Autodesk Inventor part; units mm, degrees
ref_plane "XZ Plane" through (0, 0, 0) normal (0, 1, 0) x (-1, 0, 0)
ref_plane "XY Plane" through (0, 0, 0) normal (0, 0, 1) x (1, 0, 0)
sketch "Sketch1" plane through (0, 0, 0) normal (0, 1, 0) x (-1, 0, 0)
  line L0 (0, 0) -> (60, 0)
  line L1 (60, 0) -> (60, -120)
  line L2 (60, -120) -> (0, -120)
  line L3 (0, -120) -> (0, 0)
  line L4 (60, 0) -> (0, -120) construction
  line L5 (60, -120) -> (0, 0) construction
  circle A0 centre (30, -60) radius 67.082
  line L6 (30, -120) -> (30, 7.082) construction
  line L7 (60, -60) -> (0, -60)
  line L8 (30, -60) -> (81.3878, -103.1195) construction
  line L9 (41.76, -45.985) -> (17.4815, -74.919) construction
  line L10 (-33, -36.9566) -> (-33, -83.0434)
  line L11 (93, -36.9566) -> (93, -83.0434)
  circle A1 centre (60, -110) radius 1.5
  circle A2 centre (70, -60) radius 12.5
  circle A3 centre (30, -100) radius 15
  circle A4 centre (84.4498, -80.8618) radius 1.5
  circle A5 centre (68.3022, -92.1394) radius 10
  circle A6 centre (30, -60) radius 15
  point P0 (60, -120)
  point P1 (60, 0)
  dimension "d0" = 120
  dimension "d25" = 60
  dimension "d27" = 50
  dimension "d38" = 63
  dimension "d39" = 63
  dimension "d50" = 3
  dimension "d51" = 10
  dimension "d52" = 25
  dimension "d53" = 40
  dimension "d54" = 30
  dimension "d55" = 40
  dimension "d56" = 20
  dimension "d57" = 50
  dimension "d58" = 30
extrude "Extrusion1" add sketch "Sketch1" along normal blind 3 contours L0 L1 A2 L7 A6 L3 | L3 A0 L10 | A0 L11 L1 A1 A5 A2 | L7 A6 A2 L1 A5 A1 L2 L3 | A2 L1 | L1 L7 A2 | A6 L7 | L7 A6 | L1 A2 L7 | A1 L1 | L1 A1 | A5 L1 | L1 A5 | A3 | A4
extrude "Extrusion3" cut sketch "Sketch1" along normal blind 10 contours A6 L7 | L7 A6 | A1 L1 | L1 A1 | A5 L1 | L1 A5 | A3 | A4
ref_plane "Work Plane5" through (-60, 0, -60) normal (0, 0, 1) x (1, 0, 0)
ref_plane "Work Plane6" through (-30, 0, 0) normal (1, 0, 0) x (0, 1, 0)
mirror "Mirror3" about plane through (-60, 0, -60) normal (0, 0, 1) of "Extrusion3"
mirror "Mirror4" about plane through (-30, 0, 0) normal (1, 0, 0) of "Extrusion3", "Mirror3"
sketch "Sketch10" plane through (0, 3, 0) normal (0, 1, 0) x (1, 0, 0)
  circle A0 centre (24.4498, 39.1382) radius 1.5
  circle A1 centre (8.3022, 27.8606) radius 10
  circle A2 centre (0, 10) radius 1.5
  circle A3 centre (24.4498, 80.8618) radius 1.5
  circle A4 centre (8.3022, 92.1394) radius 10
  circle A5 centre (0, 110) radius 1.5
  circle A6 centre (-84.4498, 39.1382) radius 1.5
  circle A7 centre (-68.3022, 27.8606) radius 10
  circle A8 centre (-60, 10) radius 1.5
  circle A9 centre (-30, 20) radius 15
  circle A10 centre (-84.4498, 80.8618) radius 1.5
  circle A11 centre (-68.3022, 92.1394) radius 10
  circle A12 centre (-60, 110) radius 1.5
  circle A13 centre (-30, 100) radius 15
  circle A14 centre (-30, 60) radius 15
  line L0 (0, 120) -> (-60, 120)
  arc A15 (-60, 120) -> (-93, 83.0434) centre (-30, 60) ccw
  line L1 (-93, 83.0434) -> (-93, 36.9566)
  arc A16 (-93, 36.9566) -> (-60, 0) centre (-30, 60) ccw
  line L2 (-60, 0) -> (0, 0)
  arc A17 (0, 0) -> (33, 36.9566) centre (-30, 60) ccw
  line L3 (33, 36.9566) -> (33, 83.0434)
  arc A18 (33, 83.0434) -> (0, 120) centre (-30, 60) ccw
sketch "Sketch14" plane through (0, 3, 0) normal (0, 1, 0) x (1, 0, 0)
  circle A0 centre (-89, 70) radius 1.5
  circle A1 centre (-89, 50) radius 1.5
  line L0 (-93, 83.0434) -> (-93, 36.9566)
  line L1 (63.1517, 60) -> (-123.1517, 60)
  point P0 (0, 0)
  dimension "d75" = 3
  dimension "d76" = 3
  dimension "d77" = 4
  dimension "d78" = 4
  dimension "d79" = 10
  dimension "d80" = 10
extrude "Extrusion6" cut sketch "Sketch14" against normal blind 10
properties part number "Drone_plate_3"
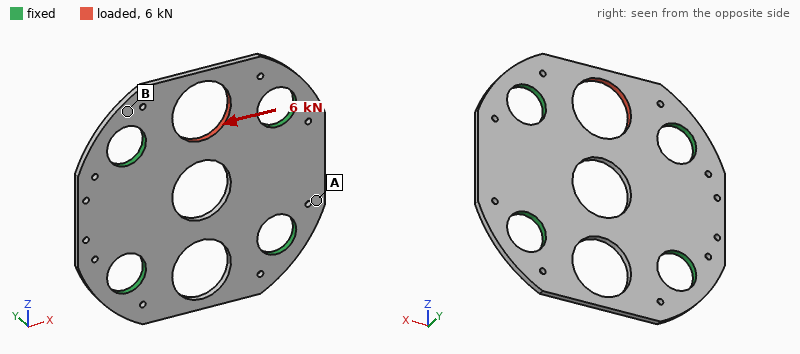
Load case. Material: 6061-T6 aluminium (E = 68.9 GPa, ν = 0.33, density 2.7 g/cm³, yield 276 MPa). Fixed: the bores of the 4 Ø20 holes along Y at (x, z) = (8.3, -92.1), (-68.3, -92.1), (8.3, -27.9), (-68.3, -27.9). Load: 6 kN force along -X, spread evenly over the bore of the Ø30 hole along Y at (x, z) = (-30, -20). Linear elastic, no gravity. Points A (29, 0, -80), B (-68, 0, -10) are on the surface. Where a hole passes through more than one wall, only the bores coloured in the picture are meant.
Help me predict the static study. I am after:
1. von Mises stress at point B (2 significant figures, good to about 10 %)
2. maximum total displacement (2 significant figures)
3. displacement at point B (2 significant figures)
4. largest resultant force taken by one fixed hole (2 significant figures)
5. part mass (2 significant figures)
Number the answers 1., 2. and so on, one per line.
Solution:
1. 23 MPa
2. 25 µm
3. 6.4 µm
4. 2.9 kN
5. 80 g
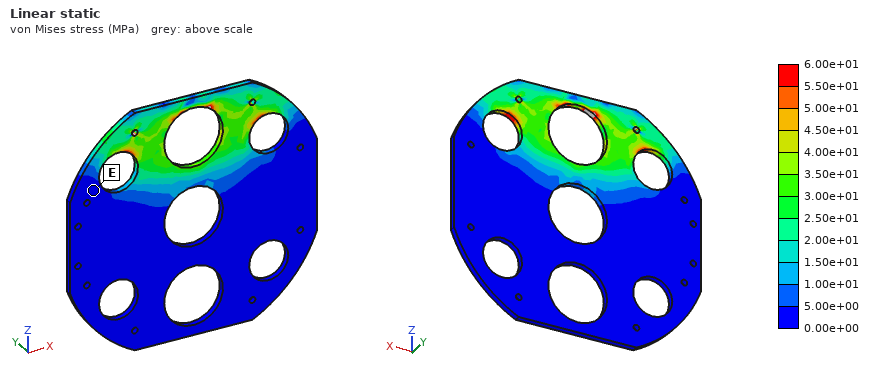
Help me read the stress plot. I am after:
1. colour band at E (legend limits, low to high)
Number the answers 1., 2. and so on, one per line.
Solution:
1. 0.00e+00 to 5.00e+00 MPa
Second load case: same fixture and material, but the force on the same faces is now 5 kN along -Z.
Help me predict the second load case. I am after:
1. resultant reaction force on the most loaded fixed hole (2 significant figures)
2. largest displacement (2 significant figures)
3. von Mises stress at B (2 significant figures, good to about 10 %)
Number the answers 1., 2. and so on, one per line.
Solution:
1. 2.1 kN
2. 44 µm
3. 7.7 MPa
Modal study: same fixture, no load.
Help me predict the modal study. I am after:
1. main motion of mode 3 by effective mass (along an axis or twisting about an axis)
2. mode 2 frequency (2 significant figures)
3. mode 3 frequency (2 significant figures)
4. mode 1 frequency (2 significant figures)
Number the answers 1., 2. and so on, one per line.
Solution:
1. along Y
2. 3500 Hz
3. 4100 Hz
4. 3500 Hz
